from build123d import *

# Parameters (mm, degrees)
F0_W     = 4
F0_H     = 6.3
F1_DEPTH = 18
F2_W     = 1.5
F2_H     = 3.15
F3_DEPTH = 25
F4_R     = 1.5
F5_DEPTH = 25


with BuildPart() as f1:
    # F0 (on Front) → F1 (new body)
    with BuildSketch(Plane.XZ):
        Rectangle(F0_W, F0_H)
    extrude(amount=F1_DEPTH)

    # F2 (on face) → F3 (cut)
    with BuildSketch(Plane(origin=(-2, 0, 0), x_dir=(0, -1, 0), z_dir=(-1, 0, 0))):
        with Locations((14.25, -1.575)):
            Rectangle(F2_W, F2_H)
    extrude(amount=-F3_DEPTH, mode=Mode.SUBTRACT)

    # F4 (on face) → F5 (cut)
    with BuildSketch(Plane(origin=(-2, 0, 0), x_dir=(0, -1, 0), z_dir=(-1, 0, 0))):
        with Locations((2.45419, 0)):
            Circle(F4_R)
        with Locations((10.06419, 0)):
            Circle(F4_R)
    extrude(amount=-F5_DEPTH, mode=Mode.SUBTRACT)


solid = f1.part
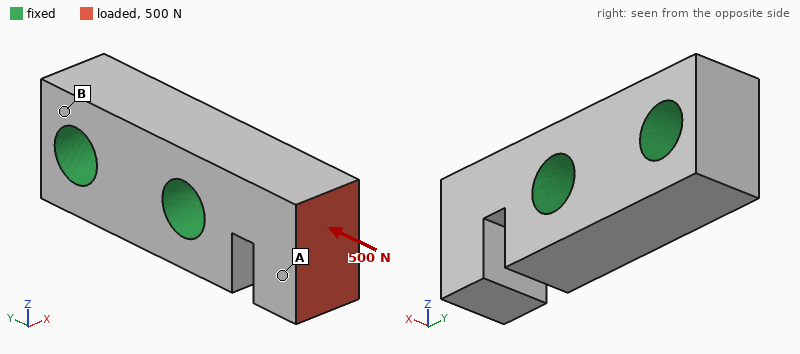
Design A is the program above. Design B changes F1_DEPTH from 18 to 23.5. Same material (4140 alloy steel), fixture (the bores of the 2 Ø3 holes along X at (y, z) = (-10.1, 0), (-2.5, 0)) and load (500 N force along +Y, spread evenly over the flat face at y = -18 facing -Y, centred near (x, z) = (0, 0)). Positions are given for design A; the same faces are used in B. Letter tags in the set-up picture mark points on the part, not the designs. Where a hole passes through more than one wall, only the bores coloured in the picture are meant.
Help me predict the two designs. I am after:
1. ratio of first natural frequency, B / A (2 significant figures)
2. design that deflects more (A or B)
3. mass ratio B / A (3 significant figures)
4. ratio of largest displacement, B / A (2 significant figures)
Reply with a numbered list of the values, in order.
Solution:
1. 0.35
2. B
3. 1.37
4. 1.5
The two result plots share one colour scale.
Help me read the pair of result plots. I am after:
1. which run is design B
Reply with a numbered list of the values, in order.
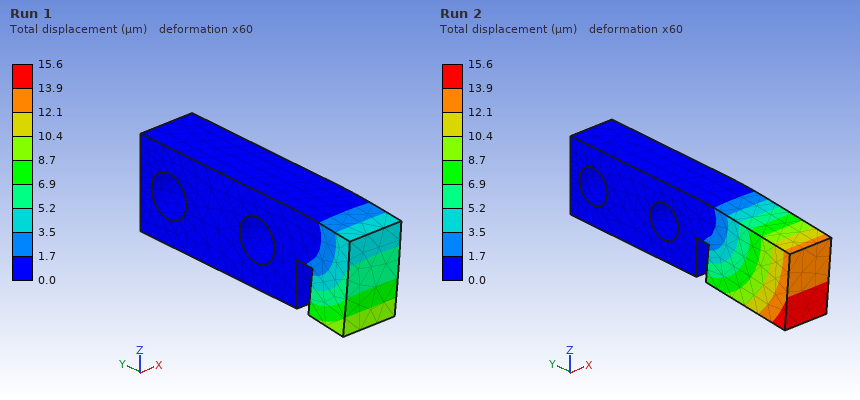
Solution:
1. Run 2
